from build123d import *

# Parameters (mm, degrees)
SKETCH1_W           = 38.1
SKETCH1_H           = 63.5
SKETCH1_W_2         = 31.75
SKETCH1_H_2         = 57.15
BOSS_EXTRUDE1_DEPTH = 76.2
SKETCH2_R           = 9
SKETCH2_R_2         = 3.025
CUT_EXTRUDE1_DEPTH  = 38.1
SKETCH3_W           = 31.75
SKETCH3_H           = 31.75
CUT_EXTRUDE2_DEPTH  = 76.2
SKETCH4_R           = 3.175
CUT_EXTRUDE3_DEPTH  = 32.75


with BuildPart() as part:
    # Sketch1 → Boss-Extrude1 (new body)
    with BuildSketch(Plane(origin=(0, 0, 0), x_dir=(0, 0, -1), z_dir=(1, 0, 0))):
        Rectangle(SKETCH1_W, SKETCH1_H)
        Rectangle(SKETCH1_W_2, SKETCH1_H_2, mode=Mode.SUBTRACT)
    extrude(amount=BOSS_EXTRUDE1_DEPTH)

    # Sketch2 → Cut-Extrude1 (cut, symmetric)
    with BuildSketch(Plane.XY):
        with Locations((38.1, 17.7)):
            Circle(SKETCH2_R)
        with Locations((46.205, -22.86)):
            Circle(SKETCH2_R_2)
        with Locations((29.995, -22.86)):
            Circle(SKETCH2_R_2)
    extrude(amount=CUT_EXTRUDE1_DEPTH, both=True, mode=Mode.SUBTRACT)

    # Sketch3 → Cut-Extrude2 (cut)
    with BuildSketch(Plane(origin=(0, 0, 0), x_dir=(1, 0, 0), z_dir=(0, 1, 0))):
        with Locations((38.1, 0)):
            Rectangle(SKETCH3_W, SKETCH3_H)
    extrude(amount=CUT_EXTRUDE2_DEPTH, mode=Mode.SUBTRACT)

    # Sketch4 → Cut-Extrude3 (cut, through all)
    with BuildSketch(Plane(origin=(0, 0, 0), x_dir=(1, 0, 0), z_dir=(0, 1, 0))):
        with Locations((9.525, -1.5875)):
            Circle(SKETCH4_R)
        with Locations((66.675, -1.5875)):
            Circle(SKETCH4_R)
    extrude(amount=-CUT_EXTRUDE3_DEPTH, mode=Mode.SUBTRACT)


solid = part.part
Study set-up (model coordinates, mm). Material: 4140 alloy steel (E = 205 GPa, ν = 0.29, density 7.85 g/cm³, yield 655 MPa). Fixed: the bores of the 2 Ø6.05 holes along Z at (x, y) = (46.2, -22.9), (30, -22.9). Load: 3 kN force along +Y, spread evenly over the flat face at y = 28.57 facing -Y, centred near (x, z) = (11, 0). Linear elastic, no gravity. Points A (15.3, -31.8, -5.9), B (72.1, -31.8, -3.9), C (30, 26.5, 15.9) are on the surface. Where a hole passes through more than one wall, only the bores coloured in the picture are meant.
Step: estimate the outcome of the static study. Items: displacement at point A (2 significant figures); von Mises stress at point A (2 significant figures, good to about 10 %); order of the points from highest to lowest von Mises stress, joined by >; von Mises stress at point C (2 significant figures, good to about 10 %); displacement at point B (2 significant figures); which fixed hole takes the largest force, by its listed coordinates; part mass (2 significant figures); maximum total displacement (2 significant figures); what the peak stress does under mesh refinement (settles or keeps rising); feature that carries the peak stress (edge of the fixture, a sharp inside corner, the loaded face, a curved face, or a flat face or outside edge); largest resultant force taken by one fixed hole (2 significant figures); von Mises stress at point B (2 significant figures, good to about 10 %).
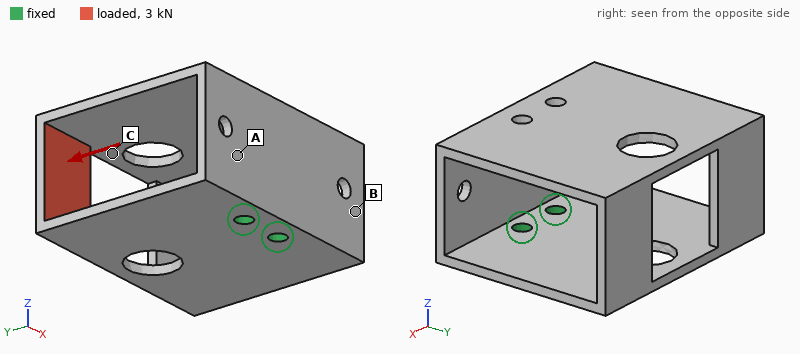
0.15 mm
130 MPa
A > B > C
34 MPa
0.13 mm
(30, -22.9)
320 g
0.81 mm
keeps rising
edge of the fixture
5.1 kN
87 MPa
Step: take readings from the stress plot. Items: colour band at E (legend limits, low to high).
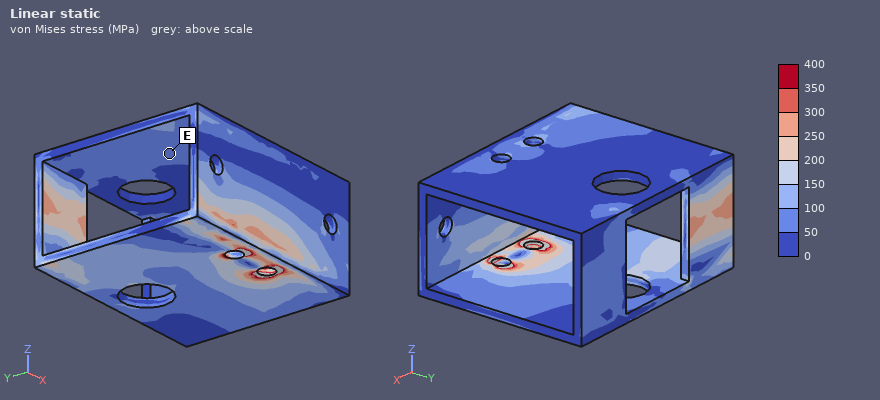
50 to 100 MPa
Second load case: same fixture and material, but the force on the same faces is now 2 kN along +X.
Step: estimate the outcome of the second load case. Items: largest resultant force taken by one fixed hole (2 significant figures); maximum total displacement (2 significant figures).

4.9 kN
0.31 mm
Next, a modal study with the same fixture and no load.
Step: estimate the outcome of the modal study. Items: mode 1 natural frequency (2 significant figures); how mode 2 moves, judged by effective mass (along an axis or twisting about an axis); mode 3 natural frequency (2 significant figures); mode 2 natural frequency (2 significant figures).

490 Hz
along X
1400 Hz
1000 Hz
